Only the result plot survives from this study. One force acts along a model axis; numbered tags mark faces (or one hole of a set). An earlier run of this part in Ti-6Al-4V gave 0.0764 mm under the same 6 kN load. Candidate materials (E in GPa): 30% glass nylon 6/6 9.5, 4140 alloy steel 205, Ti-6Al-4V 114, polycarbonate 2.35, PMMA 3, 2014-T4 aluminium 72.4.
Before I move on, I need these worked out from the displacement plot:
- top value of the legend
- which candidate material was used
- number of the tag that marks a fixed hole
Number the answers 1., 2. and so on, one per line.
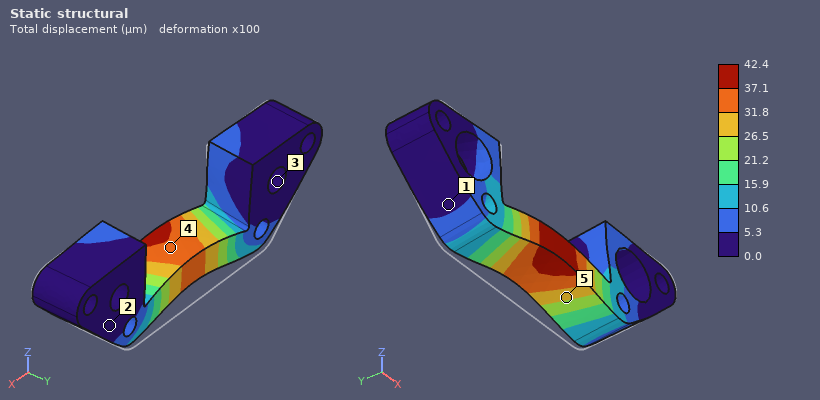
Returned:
1. 42.4 µm
2. 4140 alloy steel
3. 3
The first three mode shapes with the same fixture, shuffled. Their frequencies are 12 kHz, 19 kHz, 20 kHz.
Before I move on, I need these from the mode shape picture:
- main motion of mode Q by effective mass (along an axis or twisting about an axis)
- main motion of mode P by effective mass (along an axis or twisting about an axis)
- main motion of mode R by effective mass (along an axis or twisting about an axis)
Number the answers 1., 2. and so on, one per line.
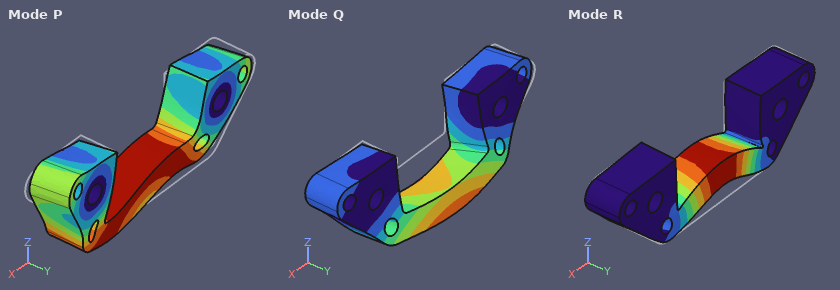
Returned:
1. along Y
2. along X
3. along Z
